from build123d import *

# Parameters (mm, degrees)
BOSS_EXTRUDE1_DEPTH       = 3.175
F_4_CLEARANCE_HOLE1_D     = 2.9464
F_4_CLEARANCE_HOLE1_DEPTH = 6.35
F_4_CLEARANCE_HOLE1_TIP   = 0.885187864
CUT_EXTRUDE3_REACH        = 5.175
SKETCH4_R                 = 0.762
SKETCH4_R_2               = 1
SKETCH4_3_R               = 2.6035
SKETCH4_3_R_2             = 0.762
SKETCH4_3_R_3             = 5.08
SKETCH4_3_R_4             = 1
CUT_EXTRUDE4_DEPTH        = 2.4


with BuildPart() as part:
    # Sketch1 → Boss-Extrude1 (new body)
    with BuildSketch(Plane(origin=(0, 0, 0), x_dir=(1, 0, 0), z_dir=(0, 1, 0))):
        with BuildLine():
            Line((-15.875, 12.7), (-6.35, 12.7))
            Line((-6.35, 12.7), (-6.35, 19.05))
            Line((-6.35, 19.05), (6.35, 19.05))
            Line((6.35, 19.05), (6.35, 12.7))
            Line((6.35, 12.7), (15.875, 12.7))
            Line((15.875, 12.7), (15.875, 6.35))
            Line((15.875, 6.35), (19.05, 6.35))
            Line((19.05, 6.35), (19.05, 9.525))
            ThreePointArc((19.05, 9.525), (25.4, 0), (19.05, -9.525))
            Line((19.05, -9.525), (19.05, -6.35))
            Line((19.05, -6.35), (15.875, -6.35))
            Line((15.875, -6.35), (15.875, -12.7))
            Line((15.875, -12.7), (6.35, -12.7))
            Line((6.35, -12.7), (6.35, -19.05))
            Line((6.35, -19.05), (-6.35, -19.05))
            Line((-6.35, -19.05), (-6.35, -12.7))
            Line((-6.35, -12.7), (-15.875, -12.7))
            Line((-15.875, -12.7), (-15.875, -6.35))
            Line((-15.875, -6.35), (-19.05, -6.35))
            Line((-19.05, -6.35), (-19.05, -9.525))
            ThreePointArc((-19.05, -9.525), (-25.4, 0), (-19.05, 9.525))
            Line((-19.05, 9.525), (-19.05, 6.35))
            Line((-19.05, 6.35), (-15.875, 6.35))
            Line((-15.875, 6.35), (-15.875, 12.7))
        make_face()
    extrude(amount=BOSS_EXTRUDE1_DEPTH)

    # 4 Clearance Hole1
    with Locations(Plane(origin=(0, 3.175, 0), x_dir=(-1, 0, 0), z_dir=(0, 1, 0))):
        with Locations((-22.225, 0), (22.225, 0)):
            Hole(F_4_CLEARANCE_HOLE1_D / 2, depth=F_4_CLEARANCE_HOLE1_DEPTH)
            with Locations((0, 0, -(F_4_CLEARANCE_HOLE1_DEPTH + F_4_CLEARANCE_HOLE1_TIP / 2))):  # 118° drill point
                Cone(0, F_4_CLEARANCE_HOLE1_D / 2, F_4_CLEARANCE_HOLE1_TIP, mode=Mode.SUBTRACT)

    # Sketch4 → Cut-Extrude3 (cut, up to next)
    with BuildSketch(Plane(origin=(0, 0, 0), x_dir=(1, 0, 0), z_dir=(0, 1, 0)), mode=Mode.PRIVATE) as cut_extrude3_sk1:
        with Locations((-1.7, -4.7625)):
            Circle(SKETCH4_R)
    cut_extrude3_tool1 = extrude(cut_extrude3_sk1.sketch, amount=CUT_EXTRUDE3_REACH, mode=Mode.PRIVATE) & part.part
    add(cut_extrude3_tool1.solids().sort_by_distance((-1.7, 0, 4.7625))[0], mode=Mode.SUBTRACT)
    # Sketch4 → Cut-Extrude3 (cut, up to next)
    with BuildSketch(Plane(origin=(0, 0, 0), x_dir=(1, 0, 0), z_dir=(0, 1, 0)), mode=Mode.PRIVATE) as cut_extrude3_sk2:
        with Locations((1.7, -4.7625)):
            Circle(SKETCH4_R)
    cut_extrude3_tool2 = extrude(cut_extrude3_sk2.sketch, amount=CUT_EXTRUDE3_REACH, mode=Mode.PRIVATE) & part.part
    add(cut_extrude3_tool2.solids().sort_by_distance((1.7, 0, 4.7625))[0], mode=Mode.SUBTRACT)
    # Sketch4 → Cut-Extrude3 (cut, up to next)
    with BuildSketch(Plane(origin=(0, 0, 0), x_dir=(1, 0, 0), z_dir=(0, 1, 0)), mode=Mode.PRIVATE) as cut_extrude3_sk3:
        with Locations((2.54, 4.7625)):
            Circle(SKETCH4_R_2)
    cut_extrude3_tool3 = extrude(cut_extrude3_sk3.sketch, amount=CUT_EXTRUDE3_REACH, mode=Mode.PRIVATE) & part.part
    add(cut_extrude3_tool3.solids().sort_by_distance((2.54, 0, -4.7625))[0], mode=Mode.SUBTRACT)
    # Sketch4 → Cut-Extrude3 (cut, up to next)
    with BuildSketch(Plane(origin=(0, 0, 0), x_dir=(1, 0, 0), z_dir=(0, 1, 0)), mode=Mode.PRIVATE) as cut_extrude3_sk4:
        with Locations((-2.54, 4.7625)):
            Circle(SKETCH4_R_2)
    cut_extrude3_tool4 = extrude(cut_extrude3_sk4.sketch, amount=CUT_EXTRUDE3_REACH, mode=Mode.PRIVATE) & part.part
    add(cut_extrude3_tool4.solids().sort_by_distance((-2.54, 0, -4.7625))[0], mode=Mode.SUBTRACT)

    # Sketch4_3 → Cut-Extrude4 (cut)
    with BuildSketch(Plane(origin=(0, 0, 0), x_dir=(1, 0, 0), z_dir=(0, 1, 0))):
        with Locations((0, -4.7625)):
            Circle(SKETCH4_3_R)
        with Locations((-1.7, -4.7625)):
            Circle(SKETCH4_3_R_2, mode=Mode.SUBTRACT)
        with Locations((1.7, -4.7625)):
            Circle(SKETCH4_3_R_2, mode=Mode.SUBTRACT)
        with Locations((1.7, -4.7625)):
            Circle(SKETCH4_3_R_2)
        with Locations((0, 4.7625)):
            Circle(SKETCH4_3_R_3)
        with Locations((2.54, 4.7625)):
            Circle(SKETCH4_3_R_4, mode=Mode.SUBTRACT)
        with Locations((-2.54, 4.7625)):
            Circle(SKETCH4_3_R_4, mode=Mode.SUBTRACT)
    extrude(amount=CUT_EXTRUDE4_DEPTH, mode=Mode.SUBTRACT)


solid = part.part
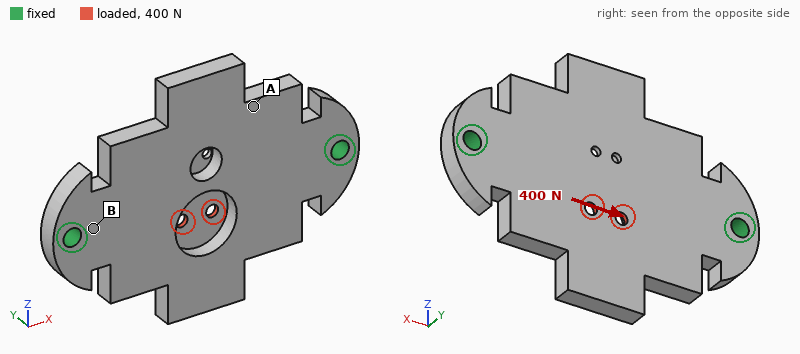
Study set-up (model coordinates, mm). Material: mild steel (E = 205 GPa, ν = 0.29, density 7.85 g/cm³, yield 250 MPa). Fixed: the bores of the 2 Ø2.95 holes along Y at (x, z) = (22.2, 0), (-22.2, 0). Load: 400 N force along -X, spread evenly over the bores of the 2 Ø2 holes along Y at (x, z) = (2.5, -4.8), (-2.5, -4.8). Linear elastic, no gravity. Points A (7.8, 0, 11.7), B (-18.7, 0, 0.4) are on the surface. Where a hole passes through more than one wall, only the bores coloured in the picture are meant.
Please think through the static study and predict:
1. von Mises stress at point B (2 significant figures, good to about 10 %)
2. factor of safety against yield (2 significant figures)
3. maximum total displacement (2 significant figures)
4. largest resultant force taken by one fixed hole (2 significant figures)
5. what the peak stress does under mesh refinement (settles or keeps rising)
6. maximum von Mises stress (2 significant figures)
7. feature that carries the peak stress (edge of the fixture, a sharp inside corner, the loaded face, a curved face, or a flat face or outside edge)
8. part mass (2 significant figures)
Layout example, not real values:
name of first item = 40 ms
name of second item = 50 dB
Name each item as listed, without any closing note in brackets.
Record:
von Mises stress at point B = 9.1 MPa
factor of safety against yield = 2.7
maximum total displacement = 1.7 µm
largest resultant force taken by one fixed hole = 210 N
what the peak stress does under mesh refinement = settles
maximum von Mises stress = 93 MPa
feature that carries the peak stress = the loaded face
part mass = 28 g
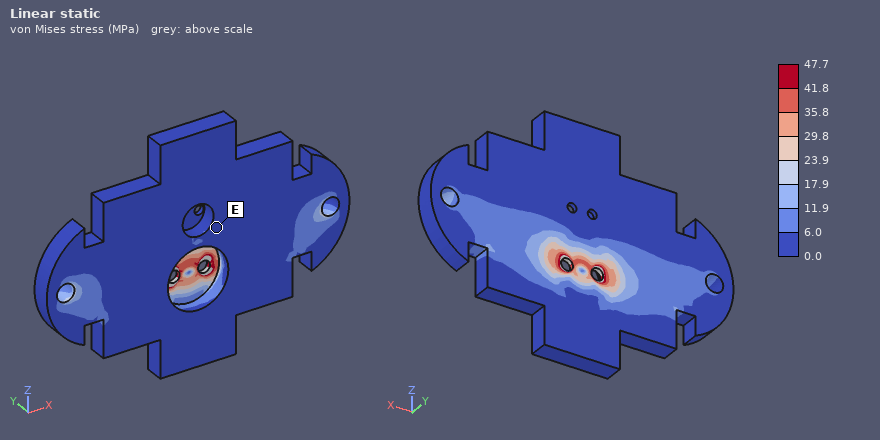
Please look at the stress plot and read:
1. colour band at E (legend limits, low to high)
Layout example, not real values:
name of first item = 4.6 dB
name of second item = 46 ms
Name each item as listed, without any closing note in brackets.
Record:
colour band at E = 0.0 to 6.0 MPa
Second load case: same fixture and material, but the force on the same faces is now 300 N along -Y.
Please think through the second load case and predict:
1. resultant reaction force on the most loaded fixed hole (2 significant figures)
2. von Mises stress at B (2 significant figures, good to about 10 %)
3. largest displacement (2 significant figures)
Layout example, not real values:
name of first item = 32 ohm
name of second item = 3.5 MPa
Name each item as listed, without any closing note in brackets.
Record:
resultant reaction force on the most loaded fixed hole = 180 N
von Mises stress at B = 59 MPa
largest displacement = 33 µm
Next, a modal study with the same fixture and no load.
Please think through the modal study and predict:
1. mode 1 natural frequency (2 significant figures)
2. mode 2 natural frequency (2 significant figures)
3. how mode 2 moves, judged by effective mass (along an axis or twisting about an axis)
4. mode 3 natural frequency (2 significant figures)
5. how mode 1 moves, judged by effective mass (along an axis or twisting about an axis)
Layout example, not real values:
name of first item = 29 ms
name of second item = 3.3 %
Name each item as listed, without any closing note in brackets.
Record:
mode 1 natural frequency = 4600 Hz
mode 2 natural frequency = 5400 Hz
how mode 2 moves, judged by effective mass = along Y
mode 3 natural frequency = 15 kHz
how mode 1 moves, judged by effective mass = twisting about X
